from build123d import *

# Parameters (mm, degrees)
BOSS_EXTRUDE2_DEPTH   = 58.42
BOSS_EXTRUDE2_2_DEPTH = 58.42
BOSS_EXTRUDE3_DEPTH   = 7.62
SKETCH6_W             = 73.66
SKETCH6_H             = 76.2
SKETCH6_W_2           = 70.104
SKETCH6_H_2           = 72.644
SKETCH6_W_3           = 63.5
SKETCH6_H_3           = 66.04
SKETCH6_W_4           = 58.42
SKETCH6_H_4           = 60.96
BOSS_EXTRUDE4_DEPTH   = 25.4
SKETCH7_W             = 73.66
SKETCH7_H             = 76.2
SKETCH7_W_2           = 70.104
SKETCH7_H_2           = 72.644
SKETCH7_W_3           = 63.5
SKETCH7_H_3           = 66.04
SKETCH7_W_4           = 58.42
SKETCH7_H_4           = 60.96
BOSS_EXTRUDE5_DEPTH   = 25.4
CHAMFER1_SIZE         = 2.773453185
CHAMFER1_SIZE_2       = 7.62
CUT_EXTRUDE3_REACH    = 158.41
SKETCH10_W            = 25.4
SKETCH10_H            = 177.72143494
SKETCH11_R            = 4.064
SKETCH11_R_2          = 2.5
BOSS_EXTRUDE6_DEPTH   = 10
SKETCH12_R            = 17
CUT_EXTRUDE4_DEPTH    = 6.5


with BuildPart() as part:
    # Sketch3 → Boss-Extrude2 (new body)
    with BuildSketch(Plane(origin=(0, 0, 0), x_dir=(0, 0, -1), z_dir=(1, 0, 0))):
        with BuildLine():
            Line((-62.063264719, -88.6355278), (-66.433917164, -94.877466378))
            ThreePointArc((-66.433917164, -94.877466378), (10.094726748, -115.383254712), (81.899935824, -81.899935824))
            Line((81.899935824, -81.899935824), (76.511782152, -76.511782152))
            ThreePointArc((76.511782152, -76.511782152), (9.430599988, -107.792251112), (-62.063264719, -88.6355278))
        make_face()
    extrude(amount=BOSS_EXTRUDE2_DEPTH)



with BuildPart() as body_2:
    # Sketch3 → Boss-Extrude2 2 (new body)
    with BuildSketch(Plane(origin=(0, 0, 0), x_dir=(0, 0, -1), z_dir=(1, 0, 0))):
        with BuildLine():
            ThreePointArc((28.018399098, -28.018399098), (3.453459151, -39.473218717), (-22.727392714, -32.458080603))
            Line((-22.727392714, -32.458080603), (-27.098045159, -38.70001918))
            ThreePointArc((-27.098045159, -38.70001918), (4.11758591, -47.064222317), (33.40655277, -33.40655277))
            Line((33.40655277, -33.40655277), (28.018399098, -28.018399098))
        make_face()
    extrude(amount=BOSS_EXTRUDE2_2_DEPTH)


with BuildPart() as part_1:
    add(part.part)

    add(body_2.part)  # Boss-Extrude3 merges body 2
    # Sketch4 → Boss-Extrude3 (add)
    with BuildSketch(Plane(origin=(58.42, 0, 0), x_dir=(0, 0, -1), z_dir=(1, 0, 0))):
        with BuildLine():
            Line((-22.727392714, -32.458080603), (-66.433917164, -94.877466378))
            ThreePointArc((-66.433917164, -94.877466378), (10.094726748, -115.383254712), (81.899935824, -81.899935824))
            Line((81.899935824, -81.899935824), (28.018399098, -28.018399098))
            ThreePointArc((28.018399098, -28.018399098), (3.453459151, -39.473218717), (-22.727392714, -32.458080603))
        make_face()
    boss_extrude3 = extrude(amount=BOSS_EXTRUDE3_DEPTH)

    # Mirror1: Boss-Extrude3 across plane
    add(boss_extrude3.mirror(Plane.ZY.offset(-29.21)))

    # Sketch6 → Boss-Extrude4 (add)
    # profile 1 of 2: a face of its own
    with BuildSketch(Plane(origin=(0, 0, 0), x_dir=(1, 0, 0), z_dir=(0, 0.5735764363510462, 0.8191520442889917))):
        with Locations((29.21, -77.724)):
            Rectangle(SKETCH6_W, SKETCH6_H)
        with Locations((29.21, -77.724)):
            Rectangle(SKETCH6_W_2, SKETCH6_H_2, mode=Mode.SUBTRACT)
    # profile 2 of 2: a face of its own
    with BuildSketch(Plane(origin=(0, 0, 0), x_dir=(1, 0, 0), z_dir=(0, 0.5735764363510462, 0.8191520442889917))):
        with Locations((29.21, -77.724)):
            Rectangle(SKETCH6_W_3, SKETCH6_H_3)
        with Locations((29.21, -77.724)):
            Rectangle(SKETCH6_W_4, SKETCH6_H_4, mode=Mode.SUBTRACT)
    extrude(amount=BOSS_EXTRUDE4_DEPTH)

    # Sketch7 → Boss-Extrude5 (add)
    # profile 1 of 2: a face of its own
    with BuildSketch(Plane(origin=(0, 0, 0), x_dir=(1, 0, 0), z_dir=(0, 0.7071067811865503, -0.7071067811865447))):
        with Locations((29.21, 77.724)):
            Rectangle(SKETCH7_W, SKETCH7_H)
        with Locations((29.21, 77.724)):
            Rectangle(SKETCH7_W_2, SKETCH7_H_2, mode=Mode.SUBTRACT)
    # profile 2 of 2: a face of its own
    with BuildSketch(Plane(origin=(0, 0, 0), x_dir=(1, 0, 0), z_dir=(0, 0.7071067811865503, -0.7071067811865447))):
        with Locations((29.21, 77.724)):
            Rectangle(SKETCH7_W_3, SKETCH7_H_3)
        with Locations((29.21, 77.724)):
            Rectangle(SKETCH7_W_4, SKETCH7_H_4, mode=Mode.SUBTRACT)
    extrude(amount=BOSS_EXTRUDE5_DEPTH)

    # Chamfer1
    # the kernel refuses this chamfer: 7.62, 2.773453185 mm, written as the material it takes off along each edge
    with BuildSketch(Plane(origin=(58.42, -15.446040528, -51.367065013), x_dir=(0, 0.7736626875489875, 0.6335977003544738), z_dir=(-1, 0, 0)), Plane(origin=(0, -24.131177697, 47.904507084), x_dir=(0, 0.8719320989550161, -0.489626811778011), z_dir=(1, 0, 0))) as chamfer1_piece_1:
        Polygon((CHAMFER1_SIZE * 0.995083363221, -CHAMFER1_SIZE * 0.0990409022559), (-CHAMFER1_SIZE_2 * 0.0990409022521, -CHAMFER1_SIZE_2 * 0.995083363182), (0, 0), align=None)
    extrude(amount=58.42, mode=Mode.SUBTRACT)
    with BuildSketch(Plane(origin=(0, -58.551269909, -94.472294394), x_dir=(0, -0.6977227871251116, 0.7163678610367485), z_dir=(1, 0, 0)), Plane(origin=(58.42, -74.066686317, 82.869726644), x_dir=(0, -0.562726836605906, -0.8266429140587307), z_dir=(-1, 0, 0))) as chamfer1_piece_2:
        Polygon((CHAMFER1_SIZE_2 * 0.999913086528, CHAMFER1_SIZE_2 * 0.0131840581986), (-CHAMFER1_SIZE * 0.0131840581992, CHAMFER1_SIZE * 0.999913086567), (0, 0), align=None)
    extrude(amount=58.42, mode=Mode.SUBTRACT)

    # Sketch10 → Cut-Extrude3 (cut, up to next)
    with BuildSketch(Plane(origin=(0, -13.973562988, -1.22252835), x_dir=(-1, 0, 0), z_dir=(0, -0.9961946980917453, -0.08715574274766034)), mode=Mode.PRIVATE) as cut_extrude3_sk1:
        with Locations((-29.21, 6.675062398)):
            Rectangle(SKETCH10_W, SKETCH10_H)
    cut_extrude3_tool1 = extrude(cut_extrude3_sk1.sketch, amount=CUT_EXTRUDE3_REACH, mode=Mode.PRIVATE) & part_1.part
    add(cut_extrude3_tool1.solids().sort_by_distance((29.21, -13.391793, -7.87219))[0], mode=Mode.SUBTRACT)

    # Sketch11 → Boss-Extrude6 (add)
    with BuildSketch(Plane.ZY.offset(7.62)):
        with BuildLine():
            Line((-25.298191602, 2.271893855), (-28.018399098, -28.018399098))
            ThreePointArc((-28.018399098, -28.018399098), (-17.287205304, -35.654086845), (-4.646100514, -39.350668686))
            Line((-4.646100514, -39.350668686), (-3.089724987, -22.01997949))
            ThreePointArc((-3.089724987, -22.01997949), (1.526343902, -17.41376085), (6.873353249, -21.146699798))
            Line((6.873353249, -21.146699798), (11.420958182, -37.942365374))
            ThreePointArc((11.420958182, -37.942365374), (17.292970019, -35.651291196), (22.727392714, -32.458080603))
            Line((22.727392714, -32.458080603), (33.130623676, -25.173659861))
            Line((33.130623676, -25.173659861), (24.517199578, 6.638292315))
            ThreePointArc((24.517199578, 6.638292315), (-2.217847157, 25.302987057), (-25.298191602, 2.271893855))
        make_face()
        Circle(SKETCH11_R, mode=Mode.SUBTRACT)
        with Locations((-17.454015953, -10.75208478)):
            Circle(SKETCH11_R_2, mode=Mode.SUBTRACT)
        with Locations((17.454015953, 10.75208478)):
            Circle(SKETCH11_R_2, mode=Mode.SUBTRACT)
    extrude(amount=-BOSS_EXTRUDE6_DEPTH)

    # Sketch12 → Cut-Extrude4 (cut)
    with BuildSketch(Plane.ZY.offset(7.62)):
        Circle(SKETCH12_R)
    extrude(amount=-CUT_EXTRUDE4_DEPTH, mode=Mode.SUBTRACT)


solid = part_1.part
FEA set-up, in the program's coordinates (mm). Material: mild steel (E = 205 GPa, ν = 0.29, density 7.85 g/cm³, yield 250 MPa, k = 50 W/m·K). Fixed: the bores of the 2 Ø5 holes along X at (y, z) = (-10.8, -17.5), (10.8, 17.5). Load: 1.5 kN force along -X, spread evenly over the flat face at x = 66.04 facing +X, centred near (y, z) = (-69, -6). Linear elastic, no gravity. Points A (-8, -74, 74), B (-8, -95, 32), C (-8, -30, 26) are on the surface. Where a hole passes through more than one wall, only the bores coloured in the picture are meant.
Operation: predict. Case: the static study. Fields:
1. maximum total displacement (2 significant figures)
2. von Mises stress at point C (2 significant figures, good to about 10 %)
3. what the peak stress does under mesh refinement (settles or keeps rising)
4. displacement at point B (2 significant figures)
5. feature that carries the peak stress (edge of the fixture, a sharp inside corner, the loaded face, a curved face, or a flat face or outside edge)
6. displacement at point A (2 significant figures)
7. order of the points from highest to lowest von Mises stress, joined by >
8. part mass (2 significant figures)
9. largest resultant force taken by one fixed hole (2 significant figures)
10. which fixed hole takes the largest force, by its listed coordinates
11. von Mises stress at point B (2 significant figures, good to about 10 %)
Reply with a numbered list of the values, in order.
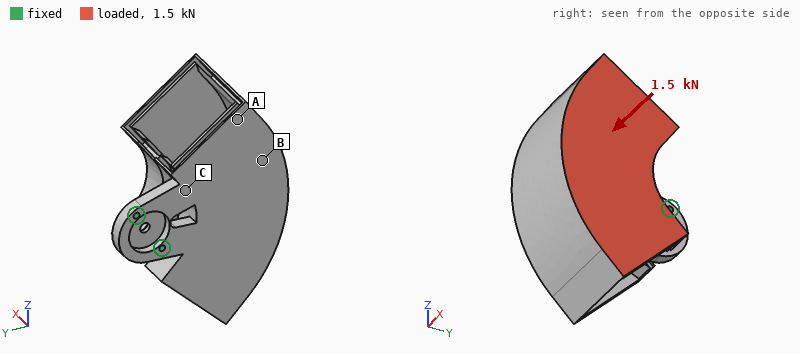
1. 0.43 mm
2. 54 MPa
3. keeps rising
4. 0.33 mm
5. edge of the fixture
6. 0.30 mm
7. C > B > A
8. 2.2 kg
9. 1.7 kN
10. (-10.8, -17.5)
11. 25 MPa
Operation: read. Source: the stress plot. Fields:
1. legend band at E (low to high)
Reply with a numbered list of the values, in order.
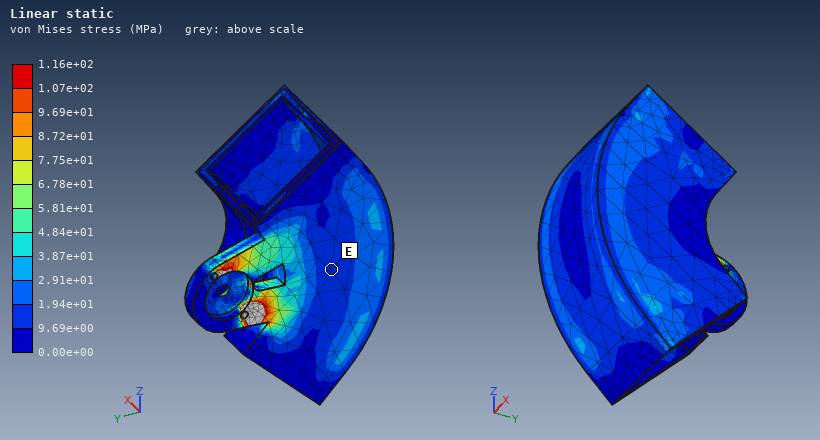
1. 9.69e+00 to 1.94e+01 MPa
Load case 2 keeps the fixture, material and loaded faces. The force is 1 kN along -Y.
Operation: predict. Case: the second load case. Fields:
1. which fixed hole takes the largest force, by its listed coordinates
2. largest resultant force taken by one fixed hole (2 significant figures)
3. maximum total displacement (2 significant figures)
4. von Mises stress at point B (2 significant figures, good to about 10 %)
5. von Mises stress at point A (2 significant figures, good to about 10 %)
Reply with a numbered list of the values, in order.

1. (-10.8, -17.5)
2. 790 N
3. 0.79 mm
4. 42 MPa
5. 20 MPa
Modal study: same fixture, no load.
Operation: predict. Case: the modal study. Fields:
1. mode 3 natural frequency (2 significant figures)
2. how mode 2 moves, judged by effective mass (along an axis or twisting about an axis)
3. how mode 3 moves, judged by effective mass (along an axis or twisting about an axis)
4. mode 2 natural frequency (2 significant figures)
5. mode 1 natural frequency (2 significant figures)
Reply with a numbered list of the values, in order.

1. 400 Hz
2. along Z
3. along X
4. 230 Hz
5. 170 Hz
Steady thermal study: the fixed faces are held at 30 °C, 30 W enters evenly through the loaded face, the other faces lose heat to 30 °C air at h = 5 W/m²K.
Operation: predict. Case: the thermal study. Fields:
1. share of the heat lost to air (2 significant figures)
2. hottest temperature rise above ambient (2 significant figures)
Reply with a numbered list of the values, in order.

1. 65 %
2. 66 K
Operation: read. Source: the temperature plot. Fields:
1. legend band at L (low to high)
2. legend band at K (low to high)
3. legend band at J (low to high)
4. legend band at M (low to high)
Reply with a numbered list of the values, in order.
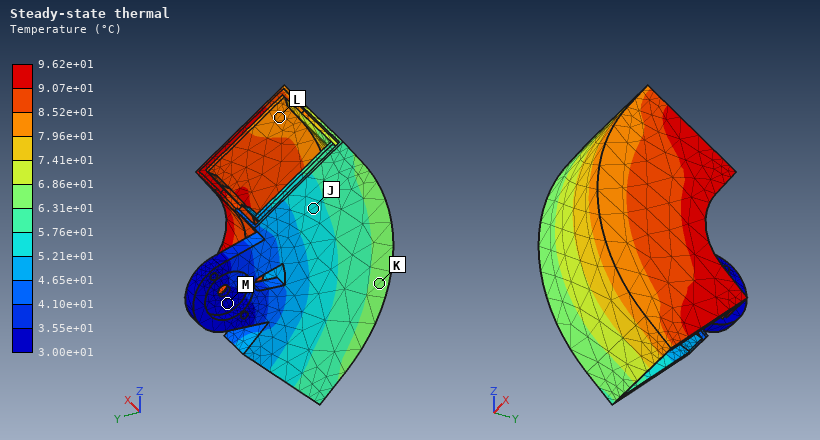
1. 7.96e+01 to 8.52e+01 °C
2. 6.31e+01 to 6.86e+01 °C
3. 5.21e+01 to 5.76e+01 °C
4. 3.00e+01 to 3.55e+01 °C
